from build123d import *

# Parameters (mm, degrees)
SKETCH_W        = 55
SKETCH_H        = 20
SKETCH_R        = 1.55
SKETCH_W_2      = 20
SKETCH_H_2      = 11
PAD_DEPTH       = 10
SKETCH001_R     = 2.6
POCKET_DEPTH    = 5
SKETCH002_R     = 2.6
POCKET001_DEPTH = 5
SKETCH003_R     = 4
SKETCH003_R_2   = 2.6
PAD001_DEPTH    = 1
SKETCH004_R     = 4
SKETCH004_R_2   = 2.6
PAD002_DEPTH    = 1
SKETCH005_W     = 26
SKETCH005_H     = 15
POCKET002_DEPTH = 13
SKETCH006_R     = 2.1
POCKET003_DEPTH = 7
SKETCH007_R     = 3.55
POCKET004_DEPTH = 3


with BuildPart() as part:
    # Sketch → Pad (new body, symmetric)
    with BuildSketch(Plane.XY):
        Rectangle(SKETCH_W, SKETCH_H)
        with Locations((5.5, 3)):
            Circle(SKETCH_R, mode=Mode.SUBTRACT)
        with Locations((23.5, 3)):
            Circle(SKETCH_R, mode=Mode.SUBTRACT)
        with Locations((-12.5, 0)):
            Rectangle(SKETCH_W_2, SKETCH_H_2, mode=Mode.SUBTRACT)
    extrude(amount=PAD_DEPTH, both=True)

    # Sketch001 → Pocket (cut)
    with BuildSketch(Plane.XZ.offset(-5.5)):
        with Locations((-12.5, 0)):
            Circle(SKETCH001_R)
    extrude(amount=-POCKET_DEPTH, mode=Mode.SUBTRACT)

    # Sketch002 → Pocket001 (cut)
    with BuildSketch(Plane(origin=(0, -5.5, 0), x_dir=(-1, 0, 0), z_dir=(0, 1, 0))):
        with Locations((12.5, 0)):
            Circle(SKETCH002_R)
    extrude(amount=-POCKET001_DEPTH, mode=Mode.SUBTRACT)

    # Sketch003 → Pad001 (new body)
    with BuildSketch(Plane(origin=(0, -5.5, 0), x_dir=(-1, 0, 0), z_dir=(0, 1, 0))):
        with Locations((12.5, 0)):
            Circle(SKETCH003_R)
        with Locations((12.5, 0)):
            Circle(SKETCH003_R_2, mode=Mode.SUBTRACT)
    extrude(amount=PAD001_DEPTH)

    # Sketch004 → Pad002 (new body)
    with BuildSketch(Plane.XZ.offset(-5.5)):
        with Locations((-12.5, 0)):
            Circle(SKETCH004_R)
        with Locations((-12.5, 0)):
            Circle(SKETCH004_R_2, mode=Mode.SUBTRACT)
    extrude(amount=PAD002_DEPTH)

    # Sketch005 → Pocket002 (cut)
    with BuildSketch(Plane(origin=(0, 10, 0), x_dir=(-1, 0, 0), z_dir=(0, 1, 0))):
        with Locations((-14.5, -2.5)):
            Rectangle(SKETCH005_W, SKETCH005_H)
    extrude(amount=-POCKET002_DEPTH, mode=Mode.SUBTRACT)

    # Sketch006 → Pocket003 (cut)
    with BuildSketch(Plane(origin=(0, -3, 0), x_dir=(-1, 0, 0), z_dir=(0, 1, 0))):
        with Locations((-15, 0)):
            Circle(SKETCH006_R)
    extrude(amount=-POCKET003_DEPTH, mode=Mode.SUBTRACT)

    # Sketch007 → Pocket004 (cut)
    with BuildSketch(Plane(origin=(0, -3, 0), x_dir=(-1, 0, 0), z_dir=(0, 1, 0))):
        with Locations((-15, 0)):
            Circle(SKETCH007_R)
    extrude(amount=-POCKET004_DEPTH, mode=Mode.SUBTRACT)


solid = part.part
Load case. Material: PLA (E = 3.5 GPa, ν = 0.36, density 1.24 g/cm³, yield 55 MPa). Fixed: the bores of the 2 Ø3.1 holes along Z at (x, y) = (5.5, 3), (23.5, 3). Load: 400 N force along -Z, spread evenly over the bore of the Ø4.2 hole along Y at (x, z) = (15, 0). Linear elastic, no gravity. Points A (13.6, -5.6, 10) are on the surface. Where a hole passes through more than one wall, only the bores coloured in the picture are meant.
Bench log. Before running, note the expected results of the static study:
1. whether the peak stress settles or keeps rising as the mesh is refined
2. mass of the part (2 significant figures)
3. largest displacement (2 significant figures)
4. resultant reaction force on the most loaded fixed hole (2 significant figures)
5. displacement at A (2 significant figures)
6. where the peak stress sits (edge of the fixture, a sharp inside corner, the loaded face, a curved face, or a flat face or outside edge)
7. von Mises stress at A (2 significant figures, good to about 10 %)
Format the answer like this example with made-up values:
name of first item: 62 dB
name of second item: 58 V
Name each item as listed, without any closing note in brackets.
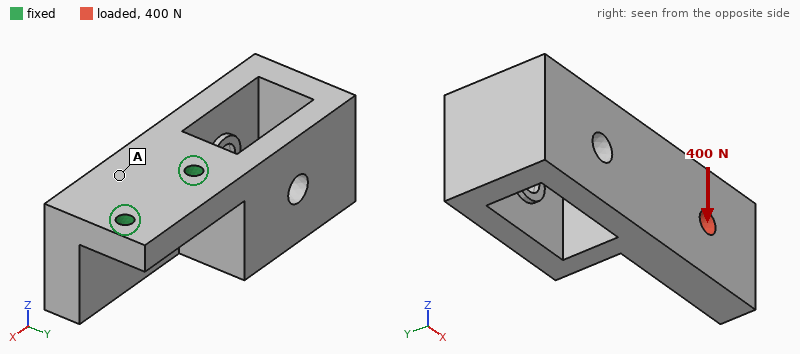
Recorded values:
whether the peak stress settles or keeps rising as the mesh is refined: keeps rising
mass of the part: 15 g
largest displacement: 0.41 mm
resultant reaction force on the most loaded fixed hole: 210 N
displacement at A: 0.14 mm
where the peak stress sits: edge of the fixture
von Mises stress at A: 5.2 MPa
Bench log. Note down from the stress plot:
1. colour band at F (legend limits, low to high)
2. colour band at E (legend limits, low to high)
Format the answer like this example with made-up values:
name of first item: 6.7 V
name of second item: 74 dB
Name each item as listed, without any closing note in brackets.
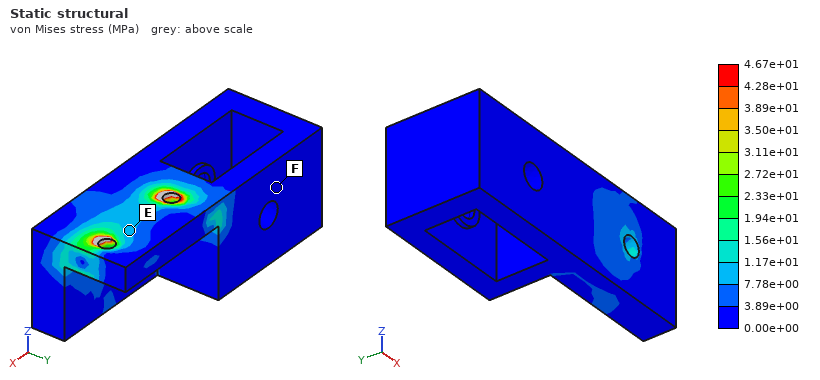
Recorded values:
colour band at F: 0.00e+00 to 3.89e+00 MPa
colour band at E: 7.78e+00 to 1.17e+01 MPa
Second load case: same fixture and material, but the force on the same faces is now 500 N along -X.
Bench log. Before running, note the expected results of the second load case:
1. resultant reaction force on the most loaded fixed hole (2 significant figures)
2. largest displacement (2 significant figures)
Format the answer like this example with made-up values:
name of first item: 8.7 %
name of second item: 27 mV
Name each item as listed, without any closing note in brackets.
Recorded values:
resultant reaction force on the most loaded fixed hole: 420 N
largest displacement: 0.25 mm
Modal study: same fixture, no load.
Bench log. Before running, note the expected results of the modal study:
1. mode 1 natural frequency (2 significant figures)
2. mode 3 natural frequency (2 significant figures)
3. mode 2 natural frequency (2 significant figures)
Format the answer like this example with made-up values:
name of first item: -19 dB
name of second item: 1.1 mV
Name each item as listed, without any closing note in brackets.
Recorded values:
mode 1 natural frequency: 1200 Hz
mode 3 natural frequency: 1900 Hz
mode 2 natural frequency: 1600 Hz
